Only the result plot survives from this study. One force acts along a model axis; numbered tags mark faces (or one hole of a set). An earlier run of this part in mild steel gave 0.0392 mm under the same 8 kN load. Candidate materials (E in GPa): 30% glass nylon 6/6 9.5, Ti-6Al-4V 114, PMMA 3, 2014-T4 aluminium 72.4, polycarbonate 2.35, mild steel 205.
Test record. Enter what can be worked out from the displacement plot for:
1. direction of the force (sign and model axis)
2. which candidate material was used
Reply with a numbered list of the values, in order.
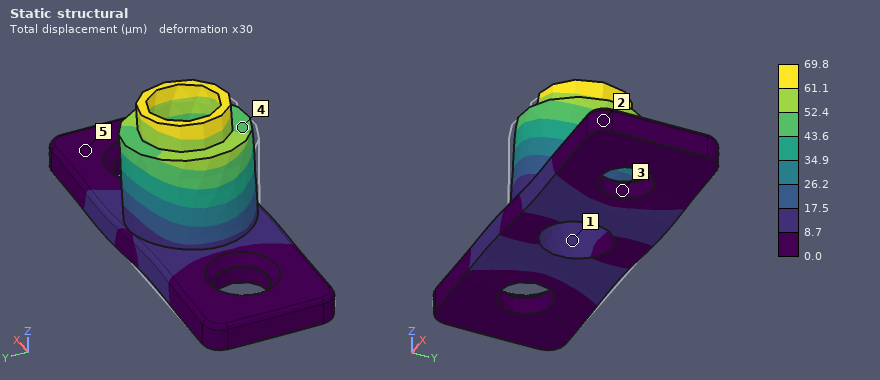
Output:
1. +X
2. Ti-6Al-4V
